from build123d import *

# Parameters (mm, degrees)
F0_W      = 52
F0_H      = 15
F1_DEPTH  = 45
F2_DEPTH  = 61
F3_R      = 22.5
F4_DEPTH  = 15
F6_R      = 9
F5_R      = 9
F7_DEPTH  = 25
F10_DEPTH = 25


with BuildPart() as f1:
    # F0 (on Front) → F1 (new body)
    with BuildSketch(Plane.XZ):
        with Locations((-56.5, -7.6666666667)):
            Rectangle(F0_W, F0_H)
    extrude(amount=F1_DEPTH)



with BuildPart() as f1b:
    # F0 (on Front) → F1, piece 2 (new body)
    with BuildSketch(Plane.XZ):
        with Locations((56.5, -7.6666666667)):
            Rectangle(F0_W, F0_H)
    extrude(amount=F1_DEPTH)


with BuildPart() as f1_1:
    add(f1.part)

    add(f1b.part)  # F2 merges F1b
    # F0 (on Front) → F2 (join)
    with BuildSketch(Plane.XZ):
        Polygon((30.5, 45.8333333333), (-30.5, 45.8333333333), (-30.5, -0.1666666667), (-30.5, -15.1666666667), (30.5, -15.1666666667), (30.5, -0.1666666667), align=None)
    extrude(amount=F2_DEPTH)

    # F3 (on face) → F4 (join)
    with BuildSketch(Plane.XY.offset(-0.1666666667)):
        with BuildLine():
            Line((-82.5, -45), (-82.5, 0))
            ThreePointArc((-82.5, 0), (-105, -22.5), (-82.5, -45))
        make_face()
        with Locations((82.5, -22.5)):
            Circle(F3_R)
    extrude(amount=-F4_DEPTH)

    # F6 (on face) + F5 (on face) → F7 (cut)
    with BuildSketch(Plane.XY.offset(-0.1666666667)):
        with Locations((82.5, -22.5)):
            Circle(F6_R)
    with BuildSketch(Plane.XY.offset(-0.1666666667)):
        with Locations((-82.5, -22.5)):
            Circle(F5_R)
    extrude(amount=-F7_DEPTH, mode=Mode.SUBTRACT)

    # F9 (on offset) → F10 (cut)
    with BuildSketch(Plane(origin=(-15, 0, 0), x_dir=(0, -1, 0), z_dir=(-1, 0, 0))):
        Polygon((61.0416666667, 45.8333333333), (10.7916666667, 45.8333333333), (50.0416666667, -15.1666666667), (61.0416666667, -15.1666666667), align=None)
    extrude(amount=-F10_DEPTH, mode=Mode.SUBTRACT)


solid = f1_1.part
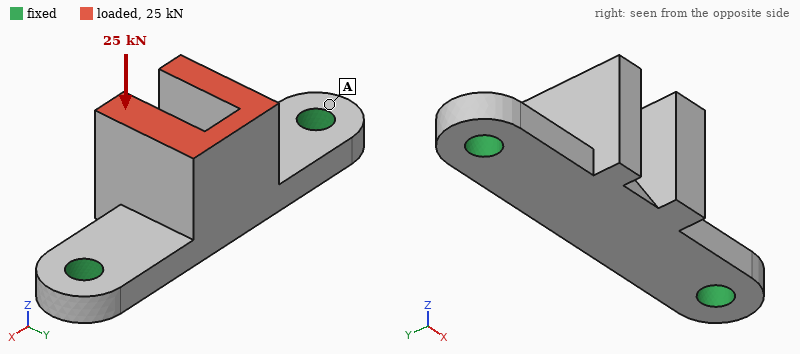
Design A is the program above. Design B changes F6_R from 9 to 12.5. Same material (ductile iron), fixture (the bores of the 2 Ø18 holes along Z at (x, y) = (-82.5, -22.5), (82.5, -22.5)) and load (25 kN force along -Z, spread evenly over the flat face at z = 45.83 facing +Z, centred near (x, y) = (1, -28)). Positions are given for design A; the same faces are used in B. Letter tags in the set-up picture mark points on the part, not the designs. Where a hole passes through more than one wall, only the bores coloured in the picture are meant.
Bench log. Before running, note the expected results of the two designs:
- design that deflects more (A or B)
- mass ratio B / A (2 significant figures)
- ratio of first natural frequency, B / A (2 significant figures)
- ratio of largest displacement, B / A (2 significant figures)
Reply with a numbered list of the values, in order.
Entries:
1. A
2. 0.99
3. 1.0
4. 0.91
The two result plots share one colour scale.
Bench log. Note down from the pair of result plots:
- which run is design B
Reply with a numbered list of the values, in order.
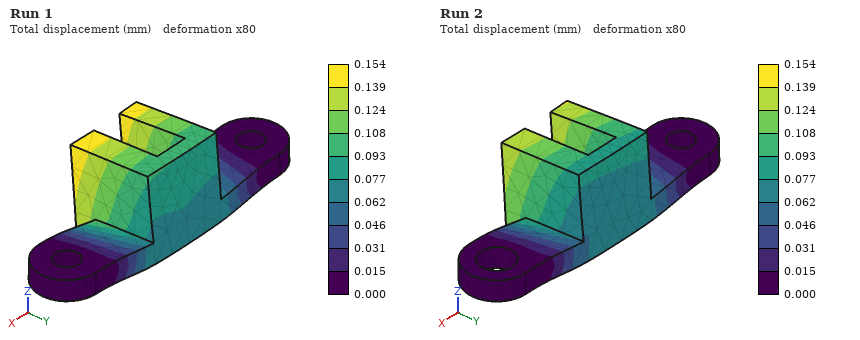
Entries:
1. Run 2
